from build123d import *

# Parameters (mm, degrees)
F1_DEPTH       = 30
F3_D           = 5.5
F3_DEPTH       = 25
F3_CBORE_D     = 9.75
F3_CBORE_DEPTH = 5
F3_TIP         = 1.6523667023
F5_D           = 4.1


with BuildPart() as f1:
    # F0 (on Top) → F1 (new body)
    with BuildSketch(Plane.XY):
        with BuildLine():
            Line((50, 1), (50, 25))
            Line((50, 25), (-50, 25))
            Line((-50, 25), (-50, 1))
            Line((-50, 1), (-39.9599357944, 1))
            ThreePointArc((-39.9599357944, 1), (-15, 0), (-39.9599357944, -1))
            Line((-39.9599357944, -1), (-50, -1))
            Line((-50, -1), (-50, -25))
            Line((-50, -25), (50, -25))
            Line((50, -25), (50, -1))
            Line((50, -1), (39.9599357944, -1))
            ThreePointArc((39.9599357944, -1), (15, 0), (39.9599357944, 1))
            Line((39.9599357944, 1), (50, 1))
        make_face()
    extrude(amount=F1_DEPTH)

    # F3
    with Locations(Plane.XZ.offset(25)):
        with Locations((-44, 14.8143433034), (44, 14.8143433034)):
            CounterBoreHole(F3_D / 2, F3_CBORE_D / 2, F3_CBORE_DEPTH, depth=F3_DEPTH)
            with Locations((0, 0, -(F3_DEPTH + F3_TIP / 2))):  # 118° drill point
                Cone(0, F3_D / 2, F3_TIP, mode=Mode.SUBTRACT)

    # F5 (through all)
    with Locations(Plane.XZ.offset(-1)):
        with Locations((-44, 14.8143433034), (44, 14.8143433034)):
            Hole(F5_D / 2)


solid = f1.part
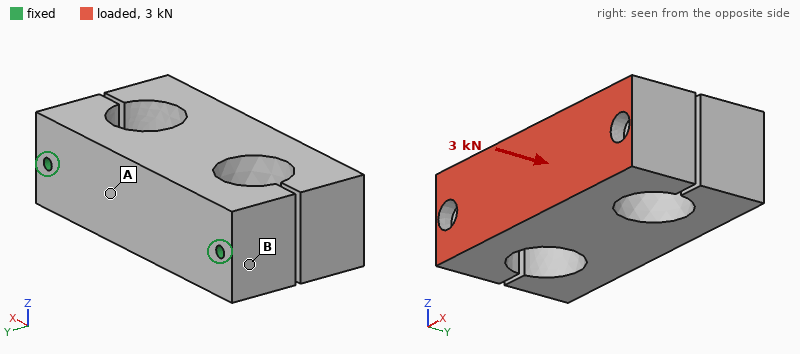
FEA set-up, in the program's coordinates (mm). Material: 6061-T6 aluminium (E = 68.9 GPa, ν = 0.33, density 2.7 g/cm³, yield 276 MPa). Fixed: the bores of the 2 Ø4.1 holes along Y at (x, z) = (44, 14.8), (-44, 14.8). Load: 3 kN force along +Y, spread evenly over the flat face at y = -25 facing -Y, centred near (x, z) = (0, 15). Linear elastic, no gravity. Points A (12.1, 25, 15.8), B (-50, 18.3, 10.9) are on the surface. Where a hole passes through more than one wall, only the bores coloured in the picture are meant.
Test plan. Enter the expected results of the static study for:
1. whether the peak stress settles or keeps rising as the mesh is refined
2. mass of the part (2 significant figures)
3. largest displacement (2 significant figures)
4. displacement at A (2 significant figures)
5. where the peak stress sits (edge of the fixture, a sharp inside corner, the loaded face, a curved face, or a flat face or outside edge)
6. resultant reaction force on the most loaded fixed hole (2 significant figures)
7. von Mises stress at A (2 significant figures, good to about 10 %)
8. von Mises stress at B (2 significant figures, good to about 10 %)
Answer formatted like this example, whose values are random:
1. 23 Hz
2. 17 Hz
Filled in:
1. keeps rising
2. 320 g
3. 33 µm
4. 12 µm
5. edge of the fixture
6. 1.5 kN
7. 11 MPa
8. 5.0 MPa
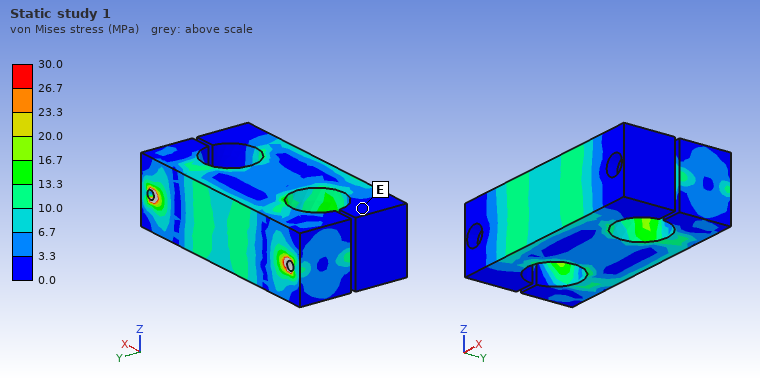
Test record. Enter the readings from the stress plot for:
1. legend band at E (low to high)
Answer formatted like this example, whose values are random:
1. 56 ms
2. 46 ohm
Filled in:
1. 0.0 to 3.3 MPa
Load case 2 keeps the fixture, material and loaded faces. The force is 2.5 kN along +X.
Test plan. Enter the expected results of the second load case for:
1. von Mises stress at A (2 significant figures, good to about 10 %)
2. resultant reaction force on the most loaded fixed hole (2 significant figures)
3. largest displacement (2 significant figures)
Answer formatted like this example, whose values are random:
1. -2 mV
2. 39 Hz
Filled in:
1. 12 MPa
2. 2.1 kN
3. 57 µm
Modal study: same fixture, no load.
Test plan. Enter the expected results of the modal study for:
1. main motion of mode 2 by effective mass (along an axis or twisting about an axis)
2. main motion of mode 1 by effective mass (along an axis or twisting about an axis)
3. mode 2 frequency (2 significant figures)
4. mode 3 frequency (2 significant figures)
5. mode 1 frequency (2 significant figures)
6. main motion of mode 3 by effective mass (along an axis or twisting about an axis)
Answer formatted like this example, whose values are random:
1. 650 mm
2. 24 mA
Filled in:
1. along X
2. along Z
3. 3200 Hz
4. 4000 Hz
5. 2000 Hz
6. twisting about Y
